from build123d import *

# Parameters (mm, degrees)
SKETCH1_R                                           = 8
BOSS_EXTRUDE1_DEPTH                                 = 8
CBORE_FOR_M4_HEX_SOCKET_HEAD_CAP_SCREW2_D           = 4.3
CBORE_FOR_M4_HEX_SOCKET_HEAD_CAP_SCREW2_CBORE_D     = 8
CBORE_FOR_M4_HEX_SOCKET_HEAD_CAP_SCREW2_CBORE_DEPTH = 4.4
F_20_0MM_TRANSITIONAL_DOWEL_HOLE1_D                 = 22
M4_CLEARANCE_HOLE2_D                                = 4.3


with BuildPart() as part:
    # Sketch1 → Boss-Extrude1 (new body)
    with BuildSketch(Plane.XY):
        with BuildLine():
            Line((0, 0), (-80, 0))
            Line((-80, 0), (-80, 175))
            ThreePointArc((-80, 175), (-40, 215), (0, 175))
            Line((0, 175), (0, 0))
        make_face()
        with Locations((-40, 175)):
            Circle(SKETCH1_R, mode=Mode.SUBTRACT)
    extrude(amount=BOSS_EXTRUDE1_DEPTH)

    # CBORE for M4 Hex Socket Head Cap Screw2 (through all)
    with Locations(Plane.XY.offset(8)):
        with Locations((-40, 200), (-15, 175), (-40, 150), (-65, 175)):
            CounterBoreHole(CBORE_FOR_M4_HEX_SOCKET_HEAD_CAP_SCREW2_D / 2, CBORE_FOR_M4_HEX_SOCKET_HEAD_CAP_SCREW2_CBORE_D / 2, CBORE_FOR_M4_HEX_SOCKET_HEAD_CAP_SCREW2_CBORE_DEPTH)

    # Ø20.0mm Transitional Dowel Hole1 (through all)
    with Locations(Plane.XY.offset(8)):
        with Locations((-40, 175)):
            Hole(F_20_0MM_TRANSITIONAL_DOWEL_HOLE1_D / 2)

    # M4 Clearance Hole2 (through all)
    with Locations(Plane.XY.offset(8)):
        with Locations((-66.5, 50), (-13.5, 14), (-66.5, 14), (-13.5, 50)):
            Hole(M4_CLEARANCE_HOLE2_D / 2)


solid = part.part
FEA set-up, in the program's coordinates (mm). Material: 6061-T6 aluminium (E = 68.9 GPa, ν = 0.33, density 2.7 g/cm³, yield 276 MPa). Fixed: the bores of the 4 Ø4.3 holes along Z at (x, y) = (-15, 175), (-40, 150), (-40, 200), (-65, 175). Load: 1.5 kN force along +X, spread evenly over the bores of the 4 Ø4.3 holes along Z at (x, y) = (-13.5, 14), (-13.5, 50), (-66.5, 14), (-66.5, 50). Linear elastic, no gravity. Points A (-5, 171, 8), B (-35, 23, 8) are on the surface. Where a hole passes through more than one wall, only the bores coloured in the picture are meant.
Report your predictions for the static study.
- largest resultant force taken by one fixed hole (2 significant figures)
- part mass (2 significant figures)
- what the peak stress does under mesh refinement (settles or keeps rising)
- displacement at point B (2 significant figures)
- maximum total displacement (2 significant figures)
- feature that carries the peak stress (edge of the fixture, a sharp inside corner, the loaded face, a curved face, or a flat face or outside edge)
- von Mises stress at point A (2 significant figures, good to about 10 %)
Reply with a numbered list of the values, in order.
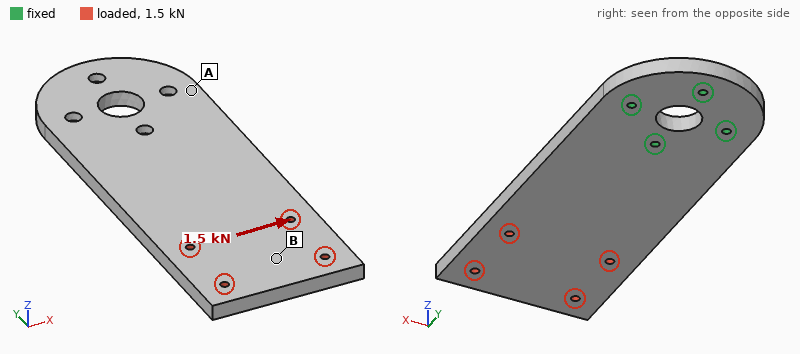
1. 2.5 kN
2. 340 g
3. keeps rising
4. 0.096 mm
5. 0.12 mm
6. edge of the fixture
7. 13 MPa
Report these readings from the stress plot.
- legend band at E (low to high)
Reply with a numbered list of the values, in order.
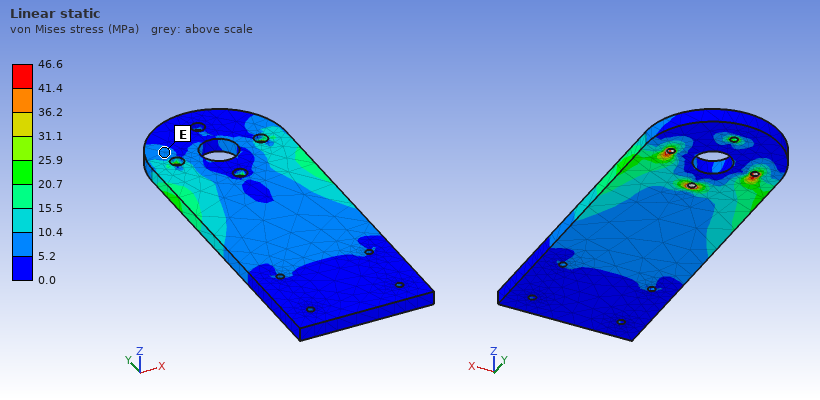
1. 5.2 to 10.4 MPa
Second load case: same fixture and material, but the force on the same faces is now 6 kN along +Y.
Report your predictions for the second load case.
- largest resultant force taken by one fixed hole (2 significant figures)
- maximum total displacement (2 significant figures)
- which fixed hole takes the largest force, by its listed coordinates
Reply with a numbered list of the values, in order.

1. 2.4 kN
2. 55 µm
3. (-40, 150)
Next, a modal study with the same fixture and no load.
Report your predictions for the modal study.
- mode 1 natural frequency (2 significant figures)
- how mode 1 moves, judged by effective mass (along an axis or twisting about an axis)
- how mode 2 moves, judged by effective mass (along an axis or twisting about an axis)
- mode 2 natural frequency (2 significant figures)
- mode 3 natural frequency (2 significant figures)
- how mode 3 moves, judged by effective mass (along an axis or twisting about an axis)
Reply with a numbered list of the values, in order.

1. 260 Hz
2. along Z
3. twisting about Y
4. 930 Hz
5. 1500 Hz
6. along Z
